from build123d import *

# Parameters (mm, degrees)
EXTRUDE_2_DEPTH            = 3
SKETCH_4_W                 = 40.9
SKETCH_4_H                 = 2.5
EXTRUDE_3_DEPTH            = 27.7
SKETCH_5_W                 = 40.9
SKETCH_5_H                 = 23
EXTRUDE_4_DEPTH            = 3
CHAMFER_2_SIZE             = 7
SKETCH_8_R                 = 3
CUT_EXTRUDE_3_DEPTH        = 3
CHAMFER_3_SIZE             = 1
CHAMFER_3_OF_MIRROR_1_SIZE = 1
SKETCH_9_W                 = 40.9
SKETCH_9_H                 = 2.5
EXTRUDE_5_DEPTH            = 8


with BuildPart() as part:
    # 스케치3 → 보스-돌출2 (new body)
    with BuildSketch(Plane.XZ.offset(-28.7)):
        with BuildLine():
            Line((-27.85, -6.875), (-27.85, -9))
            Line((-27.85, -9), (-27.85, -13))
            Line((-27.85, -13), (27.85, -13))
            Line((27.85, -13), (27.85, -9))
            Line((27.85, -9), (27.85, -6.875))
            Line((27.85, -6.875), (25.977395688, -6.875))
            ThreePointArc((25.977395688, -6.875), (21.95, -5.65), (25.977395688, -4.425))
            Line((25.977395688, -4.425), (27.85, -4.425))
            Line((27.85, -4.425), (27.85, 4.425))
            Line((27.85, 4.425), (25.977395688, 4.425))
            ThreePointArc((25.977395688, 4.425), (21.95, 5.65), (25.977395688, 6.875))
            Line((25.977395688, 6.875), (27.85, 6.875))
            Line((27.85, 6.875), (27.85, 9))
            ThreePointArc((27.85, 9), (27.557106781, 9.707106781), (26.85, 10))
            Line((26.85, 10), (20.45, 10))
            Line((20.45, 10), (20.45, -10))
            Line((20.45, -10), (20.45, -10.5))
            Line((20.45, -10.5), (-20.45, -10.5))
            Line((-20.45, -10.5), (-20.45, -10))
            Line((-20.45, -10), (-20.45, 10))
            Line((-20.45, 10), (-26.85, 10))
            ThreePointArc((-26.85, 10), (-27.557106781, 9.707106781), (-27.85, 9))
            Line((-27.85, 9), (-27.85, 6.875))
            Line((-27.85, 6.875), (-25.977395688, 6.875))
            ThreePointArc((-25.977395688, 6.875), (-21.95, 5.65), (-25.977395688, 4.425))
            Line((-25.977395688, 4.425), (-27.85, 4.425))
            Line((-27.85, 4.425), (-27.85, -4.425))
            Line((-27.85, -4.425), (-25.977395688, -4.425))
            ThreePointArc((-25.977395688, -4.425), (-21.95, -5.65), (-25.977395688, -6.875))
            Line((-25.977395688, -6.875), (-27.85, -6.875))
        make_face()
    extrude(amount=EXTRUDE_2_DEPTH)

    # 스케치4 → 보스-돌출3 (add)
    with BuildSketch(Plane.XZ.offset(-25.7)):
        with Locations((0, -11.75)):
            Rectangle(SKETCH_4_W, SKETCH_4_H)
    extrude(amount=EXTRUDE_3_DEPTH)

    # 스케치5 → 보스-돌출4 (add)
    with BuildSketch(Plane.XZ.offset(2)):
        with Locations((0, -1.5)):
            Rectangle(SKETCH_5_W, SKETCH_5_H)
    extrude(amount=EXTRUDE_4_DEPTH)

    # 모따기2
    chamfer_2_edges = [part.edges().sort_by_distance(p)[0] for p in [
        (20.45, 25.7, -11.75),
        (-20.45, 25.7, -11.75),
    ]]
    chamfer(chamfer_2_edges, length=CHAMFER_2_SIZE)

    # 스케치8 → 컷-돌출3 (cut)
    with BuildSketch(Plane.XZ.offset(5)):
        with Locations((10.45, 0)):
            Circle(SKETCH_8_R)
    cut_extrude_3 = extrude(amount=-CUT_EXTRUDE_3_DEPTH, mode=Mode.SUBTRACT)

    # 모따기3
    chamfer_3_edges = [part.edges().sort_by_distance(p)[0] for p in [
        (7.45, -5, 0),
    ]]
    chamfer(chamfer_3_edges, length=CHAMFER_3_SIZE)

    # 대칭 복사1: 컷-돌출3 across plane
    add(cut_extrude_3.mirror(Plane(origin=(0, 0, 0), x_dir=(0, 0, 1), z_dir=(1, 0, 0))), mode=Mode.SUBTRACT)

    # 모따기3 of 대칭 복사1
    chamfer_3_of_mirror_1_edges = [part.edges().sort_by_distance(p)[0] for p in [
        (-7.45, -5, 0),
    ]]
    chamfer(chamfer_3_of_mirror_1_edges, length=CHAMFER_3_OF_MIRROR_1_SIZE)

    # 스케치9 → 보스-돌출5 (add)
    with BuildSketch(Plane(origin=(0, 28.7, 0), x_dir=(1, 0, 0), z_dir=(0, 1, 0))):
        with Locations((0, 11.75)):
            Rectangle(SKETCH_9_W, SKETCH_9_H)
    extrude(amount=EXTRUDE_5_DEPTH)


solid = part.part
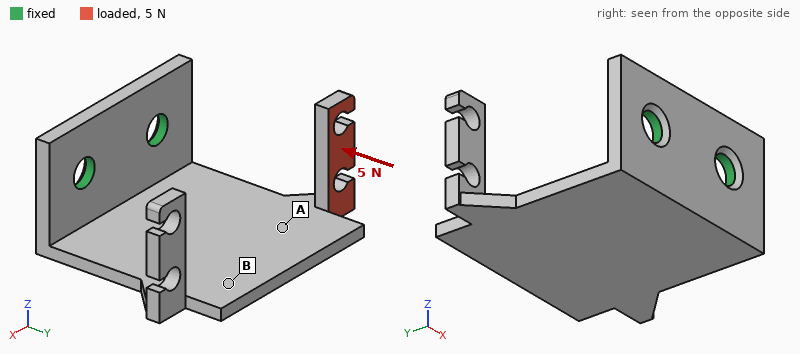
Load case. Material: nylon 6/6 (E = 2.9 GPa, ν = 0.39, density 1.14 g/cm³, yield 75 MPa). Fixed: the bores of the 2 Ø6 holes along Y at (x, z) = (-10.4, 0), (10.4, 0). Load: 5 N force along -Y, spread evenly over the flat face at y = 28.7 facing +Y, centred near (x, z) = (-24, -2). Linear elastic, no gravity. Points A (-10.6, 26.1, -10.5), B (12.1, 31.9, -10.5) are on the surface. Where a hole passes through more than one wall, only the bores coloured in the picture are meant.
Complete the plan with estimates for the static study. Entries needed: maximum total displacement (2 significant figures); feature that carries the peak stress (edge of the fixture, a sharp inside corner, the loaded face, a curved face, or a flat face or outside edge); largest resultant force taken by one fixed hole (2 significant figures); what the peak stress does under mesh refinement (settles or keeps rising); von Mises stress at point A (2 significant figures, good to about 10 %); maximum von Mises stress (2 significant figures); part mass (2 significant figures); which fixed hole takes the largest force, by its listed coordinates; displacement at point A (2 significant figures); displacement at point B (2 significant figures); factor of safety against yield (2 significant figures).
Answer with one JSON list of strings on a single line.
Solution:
["0.85 mm", "the loaded face", "7.2 N", "settles", "1.5 MPa", "16 MPa", "8.6 g", "(-10.4, 0)", "0.16 mm", "0.17 mm", "4.7"]
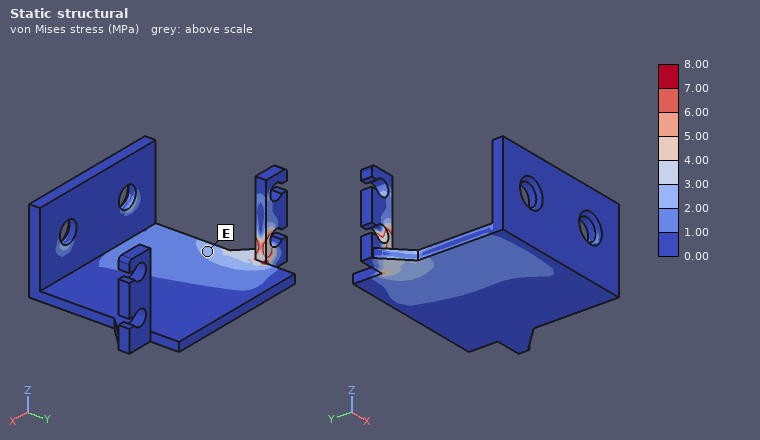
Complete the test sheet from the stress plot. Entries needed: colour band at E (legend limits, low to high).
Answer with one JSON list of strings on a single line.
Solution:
["2.00 to 3.00 MPa"]
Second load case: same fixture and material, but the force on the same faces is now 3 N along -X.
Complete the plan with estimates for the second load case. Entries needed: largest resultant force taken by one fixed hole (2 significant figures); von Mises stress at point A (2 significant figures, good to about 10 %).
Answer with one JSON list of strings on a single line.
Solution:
["4.1 N", "0.97 MPa"]
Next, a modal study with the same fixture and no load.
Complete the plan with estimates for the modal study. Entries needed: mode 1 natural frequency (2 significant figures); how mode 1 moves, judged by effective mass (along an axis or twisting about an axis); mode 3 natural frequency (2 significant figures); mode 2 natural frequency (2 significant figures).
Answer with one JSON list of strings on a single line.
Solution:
["280 Hz", "along Z", "630 Hz", "440 Hz"]
